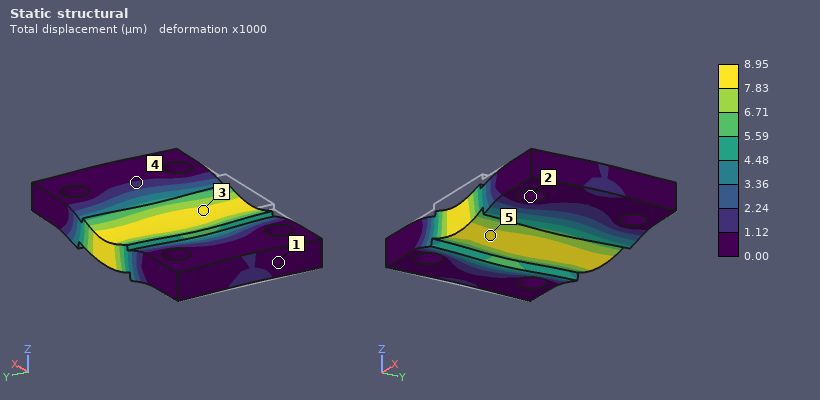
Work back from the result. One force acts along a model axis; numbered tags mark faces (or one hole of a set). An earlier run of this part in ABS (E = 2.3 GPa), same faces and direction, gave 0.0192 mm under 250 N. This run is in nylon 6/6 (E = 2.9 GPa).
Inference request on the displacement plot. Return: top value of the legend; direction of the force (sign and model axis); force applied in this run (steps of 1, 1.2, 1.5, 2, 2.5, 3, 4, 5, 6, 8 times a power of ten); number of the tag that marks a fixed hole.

8.95 µm
-Z
150 N
2
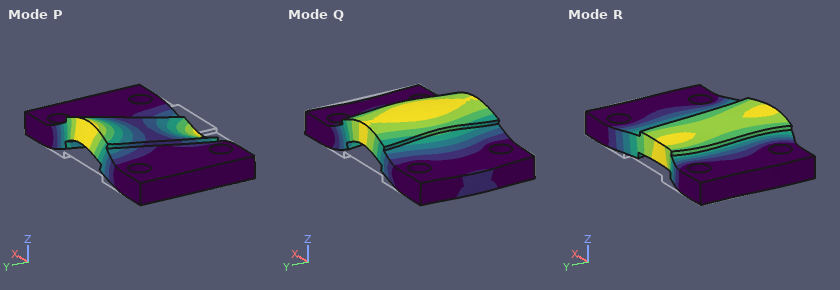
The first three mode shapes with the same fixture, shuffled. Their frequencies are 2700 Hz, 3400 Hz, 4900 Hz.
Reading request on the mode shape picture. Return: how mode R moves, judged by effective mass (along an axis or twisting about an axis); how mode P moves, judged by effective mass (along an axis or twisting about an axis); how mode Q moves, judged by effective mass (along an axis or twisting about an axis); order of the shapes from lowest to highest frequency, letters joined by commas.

along Y
twisting about X
along Z
Q, P, R
